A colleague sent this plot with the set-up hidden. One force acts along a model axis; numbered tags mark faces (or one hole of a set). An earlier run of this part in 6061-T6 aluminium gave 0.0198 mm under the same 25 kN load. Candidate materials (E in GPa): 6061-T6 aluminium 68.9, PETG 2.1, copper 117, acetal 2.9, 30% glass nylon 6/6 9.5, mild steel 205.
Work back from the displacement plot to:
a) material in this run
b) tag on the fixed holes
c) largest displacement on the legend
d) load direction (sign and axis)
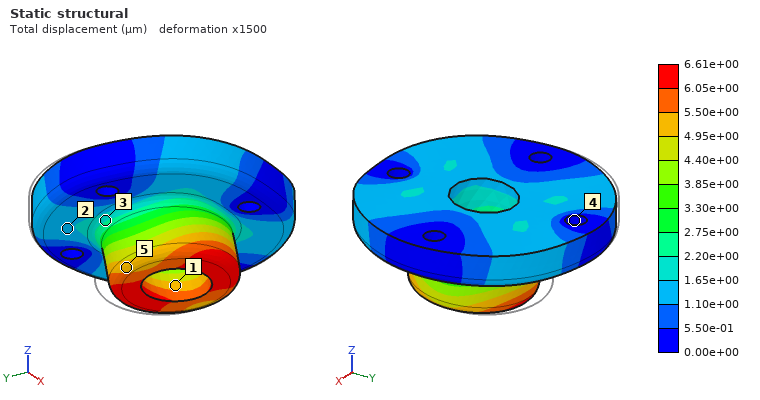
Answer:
mild steel
4
6.61e+00 µm
-Y
